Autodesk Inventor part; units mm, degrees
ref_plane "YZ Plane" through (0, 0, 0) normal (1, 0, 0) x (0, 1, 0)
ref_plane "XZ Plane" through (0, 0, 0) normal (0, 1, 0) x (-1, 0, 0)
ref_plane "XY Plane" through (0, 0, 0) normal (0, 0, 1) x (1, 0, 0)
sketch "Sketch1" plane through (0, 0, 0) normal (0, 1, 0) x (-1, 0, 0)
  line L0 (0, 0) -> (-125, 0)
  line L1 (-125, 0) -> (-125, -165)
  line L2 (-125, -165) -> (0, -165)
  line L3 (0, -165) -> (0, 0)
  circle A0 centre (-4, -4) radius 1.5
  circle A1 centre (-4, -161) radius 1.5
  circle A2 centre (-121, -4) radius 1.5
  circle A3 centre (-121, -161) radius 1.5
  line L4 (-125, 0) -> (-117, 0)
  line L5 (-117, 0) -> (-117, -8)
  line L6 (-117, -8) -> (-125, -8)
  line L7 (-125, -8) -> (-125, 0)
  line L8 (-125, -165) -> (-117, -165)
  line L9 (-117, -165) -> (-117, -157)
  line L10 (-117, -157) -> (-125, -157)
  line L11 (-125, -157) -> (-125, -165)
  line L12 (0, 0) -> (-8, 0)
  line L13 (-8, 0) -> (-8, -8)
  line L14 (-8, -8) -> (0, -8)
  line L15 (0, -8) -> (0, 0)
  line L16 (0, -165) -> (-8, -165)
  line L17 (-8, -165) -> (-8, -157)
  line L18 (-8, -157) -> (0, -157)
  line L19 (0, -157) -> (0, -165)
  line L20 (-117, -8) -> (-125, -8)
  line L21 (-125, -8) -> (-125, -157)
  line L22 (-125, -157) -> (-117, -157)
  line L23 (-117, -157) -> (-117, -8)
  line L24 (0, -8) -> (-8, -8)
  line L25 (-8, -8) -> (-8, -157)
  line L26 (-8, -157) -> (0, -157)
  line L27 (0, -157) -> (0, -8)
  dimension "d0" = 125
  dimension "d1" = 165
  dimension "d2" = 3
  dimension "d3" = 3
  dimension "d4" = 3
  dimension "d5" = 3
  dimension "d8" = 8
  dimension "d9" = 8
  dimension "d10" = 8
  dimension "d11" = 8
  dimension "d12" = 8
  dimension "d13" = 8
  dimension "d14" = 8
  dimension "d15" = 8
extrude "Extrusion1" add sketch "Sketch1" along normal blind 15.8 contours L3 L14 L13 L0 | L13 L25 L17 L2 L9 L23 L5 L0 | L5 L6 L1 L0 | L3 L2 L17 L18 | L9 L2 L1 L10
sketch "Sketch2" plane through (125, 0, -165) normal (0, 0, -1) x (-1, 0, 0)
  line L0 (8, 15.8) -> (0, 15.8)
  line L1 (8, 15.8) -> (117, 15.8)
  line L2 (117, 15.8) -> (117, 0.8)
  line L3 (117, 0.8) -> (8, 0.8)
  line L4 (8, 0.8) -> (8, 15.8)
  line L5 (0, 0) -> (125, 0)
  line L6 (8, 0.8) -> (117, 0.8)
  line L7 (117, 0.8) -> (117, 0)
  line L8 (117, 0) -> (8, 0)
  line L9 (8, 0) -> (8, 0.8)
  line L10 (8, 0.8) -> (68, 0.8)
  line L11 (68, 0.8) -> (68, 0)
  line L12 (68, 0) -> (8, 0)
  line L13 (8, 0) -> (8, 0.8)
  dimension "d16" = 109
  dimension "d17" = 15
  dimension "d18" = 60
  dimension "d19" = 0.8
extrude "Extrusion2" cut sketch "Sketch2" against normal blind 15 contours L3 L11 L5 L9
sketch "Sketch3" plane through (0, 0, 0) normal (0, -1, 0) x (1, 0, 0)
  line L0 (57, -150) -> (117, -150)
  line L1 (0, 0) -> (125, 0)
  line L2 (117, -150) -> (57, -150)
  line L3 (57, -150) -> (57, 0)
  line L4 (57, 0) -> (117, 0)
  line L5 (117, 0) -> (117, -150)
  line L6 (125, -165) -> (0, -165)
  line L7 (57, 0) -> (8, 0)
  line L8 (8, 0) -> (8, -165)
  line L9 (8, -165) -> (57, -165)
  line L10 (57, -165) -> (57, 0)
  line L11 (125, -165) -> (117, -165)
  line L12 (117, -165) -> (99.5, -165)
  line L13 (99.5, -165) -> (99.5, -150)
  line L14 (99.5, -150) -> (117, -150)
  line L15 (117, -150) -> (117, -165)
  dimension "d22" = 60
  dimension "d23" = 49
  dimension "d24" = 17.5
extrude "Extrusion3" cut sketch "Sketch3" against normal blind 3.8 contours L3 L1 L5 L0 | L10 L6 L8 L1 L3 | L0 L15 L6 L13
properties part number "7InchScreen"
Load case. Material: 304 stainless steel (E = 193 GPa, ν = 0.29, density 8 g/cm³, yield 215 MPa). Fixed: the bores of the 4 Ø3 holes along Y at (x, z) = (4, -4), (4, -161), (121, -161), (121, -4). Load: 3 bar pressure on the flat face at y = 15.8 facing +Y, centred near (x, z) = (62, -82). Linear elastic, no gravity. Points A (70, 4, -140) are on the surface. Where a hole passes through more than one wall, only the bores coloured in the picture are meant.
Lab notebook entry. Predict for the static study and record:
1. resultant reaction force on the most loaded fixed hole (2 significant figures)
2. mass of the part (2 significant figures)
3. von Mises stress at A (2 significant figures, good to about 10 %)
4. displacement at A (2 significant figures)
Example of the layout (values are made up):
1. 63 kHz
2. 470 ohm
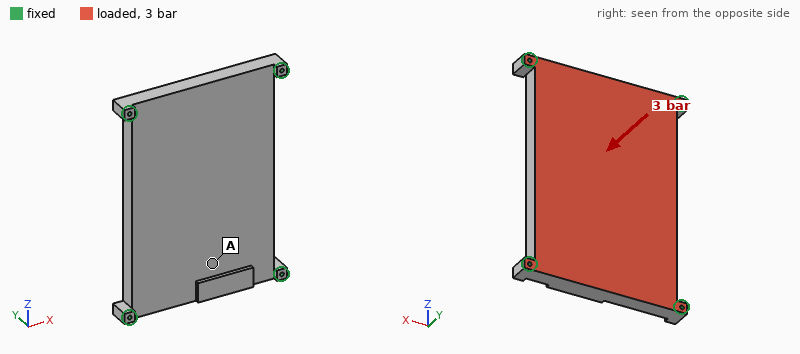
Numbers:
1. 1.4 kN
2. 1.8 kg
3. 10 MPa
4. 31 µm
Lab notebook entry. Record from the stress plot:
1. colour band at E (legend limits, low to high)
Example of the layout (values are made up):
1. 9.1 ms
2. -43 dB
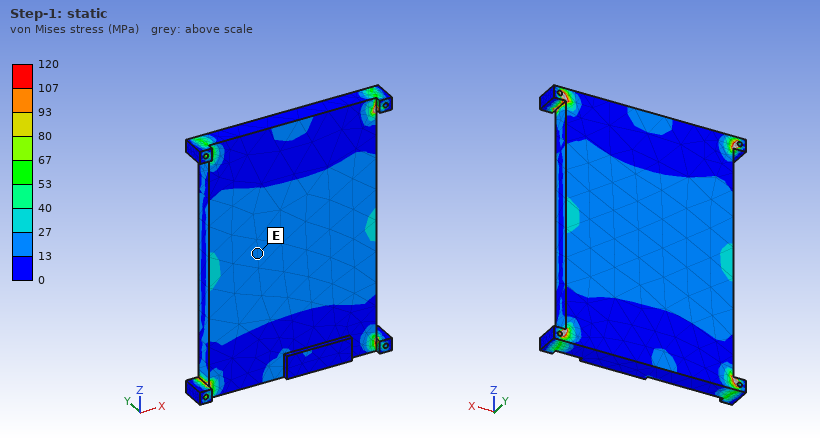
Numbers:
1. 13 to 27 MPa
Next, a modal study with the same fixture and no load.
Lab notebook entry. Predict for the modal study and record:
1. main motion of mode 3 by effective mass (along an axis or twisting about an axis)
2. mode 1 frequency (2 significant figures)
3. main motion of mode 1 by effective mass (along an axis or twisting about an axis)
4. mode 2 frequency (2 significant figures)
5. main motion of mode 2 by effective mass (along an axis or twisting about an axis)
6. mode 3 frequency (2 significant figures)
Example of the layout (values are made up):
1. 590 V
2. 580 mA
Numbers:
1. twisting about X
2. 1300 Hz
3. along Y
4. 2600 Hz
5. twisting about Z
6. 3300 Hz
